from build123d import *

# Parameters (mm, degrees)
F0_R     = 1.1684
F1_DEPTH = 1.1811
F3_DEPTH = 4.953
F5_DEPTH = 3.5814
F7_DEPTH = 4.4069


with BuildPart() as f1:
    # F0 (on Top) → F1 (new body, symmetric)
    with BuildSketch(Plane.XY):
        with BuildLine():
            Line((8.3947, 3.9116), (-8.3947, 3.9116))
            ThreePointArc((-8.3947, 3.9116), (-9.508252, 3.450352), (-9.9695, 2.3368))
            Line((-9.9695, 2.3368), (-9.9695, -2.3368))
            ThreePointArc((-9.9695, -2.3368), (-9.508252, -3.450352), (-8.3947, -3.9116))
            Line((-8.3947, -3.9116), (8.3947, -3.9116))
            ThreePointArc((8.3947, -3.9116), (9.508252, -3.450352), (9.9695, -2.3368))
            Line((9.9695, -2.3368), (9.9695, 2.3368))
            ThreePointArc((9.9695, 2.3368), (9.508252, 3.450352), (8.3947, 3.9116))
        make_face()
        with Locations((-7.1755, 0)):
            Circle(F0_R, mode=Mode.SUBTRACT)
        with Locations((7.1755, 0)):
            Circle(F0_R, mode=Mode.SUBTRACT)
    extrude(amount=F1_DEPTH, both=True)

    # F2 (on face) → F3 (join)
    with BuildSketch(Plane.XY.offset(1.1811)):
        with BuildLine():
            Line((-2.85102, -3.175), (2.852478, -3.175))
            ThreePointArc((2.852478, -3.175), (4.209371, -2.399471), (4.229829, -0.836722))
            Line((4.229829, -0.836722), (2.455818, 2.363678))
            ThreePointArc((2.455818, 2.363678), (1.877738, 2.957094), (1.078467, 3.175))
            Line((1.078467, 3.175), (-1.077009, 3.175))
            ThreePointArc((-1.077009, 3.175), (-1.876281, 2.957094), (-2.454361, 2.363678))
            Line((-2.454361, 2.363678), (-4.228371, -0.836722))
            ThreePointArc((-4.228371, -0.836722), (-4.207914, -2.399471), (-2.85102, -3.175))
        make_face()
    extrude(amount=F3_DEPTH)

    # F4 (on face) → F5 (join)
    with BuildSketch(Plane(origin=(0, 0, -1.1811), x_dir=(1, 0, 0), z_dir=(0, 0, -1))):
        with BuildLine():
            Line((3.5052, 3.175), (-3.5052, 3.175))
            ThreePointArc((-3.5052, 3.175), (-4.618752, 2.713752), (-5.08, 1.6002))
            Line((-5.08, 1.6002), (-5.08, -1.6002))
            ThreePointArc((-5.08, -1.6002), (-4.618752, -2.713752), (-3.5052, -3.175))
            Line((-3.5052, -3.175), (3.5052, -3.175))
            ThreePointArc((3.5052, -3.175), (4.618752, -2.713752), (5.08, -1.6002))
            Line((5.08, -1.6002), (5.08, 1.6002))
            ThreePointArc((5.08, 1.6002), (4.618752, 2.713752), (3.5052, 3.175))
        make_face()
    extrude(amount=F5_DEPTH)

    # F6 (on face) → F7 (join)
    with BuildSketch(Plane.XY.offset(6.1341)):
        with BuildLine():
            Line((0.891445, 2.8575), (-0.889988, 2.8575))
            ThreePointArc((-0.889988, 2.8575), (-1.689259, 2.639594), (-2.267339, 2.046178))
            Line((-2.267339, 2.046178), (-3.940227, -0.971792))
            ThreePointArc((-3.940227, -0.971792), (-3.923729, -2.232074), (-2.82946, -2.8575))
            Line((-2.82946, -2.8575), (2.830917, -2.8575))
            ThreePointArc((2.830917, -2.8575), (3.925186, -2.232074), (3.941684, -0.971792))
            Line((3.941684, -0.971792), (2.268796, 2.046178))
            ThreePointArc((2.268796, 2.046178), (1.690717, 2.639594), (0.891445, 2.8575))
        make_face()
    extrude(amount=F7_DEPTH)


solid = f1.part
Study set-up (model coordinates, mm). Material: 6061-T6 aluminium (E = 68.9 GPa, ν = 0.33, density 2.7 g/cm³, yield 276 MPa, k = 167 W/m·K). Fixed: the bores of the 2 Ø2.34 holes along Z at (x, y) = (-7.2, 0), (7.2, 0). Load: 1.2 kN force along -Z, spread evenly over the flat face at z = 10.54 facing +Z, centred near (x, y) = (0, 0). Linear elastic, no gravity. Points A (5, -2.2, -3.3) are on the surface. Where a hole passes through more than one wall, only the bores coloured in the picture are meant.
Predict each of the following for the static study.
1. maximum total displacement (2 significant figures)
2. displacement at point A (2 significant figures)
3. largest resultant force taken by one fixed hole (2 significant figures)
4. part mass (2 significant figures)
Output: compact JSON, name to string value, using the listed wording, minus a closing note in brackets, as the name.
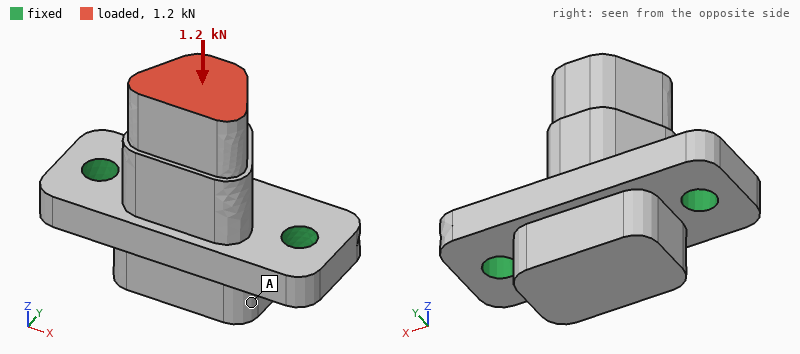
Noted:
{"maximum total displacement": "14 µm", "displacement at point A": "7.3 µm", "largest resultant force taken by one fixed hole": "600 N", "part mass": "2.6 g"}
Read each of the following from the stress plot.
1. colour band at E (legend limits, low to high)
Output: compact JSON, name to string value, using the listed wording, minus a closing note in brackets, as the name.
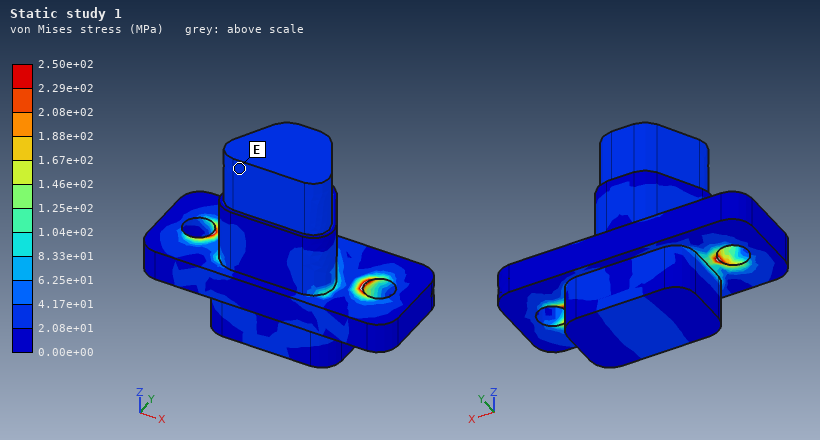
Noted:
{"colour band at E": "2.08e+01 to 4.17e+01 MPa"}
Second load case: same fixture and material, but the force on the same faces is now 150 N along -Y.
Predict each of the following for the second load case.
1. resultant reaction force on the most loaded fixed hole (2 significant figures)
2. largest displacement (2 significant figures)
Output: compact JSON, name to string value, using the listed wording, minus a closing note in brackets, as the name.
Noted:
{"resultant reaction force on the most loaded fixed hole": "76 N", "largest displacement": "36 µm"}
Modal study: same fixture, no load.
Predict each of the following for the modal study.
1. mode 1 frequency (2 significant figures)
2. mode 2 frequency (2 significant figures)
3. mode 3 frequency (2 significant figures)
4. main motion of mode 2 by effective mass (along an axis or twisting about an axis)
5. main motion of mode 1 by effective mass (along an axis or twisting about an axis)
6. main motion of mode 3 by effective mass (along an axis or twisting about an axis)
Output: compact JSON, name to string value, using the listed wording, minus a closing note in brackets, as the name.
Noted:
{"mode 1 frequency": "16 kHz", "mode 2 frequency": "34 kHz", "mode 3 frequency": "43 kHz", "main motion of mode 2 by effective mass": "along X", "main motion of mode 1 by effective mass": "along Y", "main motion of mode 3 by effective mass": "along Z"}
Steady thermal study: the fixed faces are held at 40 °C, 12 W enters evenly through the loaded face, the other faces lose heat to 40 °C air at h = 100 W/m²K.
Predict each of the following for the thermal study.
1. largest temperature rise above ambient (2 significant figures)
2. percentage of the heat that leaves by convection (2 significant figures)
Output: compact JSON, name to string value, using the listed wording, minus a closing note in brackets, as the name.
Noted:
{"largest temperature rise above ambient": "25 K", "percentage of the heat that leaves by convection": "4.6 %"}
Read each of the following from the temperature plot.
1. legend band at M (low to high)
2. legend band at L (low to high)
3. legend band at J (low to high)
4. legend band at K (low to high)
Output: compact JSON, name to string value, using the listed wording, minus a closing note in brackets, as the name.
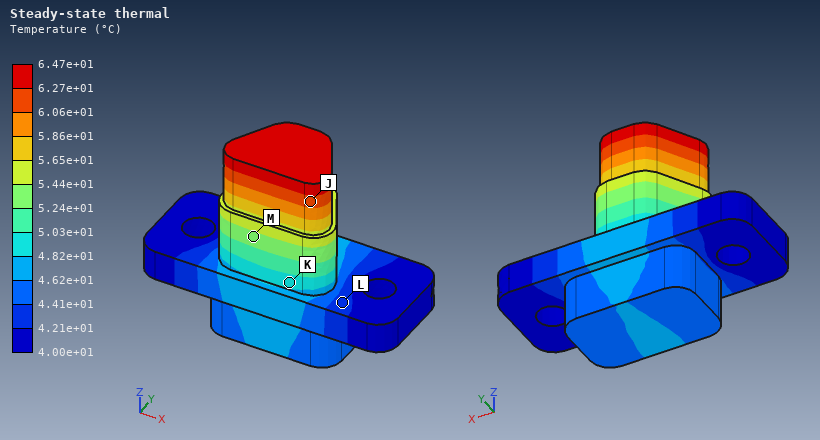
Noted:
{"legend band at M": "5.24e+01 to 5.44e+01 °C", "legend band at L": "4.21e+01 to 4.41e+01 °C", "legend band at J": "6.06e+01 to 6.27e+01 °C", "legend band at K": "4.82e+01 to 5.03e+01 °C"}
